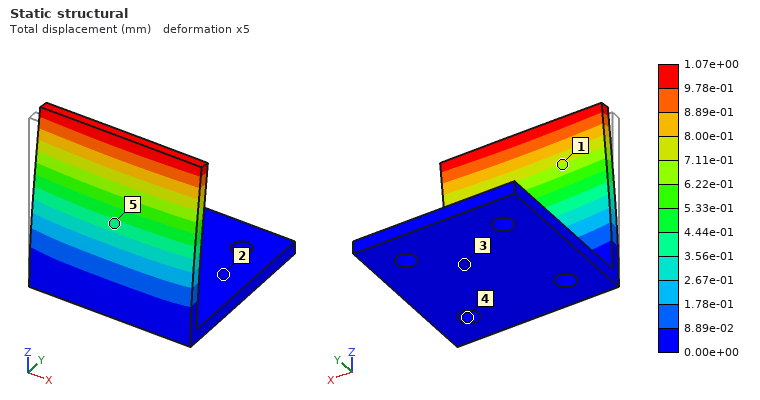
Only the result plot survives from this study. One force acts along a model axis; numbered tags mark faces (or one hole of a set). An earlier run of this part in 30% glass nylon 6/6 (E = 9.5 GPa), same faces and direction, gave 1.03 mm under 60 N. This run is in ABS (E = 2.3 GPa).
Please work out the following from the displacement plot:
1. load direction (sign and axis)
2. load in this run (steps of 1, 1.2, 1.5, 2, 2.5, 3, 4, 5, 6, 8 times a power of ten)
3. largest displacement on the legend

+Y
15 N
1.07e+00 mm
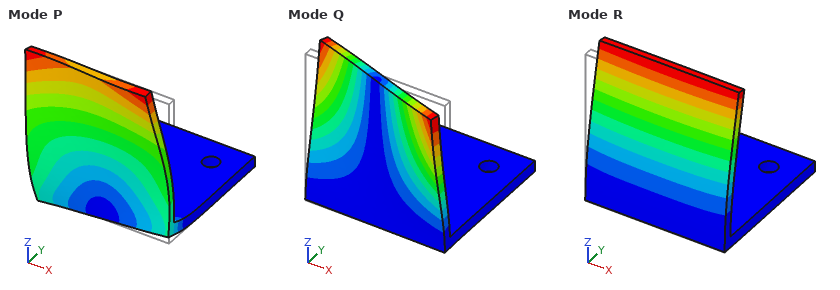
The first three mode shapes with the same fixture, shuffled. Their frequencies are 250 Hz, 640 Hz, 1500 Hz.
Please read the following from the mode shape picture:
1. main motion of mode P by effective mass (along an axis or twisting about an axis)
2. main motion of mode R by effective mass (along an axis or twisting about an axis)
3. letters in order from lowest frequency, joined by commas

along X
along Y
R, Q, P
